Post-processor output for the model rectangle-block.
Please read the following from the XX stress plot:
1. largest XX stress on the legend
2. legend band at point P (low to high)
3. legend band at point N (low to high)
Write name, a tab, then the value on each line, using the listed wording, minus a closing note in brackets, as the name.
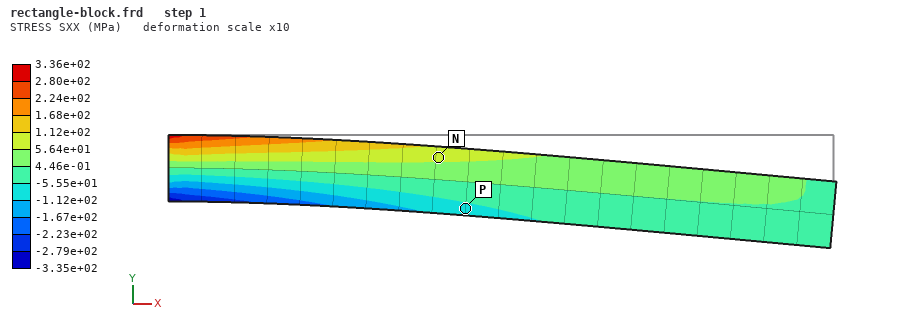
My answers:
largest XX stress on the legend	3.36e+02 MPa
legend band at point P	-1.12e+02 to -5.55e+01 MPa
legend band at point N	5.64e+01 to 1.12e+02 MPa
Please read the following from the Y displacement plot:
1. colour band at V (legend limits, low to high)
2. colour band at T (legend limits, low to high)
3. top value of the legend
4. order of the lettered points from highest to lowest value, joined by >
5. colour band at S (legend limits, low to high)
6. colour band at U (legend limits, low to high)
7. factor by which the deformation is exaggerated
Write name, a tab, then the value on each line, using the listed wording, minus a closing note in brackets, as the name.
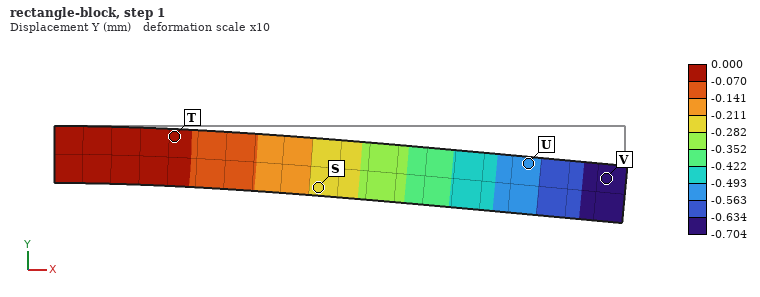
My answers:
colour band at V	-0.704 to -0.634 mm
colour band at T	-0.070 to 0.000 mm
top value of the legend	0.000 mm
order of the lettered points from highest to lowest value, joined by >	T > S > U > V
colour band at S	-0.282 to -0.211 mm
colour band at U	-0.563 to -0.493 mm
factor by which the deformation is exaggerated	10
